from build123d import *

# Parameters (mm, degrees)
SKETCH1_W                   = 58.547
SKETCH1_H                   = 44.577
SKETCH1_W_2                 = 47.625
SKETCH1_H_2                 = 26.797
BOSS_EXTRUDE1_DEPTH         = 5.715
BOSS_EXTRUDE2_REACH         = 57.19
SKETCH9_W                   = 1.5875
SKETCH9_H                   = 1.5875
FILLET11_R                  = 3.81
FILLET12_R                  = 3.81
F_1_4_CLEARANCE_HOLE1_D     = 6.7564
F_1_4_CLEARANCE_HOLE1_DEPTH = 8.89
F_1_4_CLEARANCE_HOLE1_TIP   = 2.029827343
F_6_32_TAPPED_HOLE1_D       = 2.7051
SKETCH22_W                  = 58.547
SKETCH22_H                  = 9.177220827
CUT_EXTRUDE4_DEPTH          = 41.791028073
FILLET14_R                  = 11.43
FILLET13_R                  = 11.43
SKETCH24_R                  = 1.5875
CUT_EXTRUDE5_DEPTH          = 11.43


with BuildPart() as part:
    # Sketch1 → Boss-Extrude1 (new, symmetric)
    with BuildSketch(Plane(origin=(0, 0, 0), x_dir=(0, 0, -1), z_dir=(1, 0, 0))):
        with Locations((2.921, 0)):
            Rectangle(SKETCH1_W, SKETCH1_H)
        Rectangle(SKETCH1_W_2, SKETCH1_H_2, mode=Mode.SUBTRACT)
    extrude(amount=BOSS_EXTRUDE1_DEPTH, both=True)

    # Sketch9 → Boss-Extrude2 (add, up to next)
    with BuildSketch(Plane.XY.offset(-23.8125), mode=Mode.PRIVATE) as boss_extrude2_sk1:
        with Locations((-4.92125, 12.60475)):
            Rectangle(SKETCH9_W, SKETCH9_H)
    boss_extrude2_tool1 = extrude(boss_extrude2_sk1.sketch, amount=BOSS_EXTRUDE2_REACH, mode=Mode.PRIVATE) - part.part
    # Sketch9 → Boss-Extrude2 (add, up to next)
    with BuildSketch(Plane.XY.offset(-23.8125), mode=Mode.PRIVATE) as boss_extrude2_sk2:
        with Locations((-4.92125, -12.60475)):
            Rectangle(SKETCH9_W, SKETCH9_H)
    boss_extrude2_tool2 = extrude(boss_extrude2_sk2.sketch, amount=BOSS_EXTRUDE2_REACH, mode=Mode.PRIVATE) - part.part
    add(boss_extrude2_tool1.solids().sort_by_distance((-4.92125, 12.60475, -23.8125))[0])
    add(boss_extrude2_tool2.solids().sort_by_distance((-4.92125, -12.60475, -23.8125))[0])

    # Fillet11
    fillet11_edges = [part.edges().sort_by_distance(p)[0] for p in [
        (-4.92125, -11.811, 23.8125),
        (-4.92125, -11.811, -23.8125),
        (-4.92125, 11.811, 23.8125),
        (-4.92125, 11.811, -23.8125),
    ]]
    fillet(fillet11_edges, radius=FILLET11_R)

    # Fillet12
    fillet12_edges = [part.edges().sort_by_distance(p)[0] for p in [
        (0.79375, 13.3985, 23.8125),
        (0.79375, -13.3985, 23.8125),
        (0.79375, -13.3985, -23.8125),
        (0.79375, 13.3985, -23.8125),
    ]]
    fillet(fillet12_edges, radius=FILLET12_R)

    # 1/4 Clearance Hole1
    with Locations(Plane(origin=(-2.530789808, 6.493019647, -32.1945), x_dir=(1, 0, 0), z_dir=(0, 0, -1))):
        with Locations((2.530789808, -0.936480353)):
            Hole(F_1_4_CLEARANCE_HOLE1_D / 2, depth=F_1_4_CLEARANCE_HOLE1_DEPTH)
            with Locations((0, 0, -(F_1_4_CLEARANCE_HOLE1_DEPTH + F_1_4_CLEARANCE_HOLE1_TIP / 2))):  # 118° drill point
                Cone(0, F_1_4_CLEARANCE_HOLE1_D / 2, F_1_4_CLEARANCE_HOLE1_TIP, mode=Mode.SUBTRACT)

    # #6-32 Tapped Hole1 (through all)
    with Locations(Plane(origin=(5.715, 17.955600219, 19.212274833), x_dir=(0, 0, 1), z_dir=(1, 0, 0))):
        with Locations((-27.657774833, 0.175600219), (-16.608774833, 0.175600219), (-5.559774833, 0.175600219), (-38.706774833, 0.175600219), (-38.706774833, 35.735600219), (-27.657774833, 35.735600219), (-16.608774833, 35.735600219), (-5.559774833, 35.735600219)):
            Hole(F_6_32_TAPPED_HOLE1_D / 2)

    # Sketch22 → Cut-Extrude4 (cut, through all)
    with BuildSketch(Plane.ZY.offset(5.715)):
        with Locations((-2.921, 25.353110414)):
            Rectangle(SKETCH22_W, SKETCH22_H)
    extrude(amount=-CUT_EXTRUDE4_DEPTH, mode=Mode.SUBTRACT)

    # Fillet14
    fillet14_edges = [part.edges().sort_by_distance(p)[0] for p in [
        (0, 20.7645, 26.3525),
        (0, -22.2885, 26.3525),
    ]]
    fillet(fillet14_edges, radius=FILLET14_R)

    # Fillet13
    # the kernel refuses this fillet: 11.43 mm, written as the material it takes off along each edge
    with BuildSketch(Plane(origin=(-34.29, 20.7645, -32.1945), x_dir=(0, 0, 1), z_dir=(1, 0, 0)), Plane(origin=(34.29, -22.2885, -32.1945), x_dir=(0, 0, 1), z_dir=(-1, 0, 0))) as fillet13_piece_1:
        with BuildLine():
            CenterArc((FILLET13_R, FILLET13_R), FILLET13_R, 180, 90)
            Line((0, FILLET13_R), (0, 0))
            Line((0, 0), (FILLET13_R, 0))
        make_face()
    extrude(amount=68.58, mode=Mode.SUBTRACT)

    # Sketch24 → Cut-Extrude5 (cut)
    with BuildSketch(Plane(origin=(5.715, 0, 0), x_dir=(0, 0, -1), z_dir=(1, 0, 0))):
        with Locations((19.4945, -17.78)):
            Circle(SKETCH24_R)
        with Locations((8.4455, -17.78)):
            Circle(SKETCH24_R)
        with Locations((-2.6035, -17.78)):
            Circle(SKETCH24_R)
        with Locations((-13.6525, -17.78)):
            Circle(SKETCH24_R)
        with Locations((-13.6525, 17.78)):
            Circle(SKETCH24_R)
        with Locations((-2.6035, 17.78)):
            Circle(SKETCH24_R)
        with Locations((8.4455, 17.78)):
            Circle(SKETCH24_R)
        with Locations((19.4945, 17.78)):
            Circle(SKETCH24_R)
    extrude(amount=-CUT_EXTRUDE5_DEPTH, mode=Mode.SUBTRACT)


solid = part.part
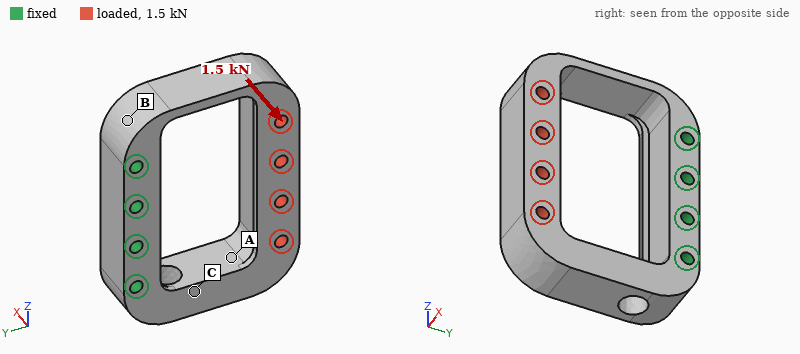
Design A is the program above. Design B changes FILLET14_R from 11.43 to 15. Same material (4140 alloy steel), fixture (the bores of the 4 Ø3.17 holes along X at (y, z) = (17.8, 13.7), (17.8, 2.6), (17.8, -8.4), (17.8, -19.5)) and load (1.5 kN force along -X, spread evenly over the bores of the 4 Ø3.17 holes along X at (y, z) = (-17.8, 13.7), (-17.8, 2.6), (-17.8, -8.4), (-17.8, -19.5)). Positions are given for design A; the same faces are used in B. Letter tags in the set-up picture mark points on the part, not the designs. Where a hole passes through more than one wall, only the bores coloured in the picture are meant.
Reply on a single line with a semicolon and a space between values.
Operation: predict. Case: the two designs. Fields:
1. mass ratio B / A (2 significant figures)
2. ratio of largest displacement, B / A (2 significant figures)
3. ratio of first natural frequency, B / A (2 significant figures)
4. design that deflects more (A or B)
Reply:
0.96; 1.2; 0.95; B
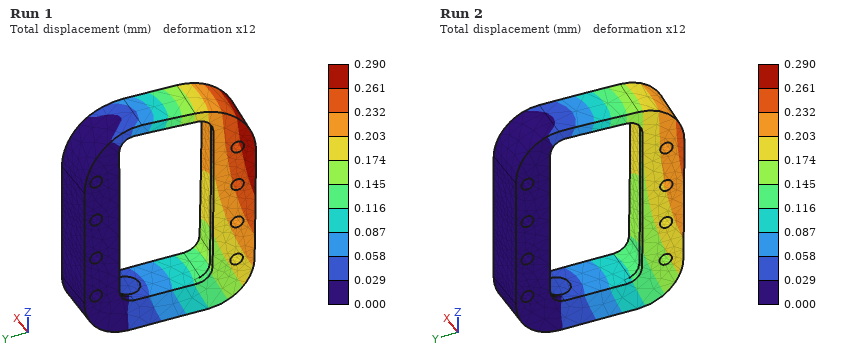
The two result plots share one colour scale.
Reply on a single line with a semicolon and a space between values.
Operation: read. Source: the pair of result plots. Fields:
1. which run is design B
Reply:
Run 1
